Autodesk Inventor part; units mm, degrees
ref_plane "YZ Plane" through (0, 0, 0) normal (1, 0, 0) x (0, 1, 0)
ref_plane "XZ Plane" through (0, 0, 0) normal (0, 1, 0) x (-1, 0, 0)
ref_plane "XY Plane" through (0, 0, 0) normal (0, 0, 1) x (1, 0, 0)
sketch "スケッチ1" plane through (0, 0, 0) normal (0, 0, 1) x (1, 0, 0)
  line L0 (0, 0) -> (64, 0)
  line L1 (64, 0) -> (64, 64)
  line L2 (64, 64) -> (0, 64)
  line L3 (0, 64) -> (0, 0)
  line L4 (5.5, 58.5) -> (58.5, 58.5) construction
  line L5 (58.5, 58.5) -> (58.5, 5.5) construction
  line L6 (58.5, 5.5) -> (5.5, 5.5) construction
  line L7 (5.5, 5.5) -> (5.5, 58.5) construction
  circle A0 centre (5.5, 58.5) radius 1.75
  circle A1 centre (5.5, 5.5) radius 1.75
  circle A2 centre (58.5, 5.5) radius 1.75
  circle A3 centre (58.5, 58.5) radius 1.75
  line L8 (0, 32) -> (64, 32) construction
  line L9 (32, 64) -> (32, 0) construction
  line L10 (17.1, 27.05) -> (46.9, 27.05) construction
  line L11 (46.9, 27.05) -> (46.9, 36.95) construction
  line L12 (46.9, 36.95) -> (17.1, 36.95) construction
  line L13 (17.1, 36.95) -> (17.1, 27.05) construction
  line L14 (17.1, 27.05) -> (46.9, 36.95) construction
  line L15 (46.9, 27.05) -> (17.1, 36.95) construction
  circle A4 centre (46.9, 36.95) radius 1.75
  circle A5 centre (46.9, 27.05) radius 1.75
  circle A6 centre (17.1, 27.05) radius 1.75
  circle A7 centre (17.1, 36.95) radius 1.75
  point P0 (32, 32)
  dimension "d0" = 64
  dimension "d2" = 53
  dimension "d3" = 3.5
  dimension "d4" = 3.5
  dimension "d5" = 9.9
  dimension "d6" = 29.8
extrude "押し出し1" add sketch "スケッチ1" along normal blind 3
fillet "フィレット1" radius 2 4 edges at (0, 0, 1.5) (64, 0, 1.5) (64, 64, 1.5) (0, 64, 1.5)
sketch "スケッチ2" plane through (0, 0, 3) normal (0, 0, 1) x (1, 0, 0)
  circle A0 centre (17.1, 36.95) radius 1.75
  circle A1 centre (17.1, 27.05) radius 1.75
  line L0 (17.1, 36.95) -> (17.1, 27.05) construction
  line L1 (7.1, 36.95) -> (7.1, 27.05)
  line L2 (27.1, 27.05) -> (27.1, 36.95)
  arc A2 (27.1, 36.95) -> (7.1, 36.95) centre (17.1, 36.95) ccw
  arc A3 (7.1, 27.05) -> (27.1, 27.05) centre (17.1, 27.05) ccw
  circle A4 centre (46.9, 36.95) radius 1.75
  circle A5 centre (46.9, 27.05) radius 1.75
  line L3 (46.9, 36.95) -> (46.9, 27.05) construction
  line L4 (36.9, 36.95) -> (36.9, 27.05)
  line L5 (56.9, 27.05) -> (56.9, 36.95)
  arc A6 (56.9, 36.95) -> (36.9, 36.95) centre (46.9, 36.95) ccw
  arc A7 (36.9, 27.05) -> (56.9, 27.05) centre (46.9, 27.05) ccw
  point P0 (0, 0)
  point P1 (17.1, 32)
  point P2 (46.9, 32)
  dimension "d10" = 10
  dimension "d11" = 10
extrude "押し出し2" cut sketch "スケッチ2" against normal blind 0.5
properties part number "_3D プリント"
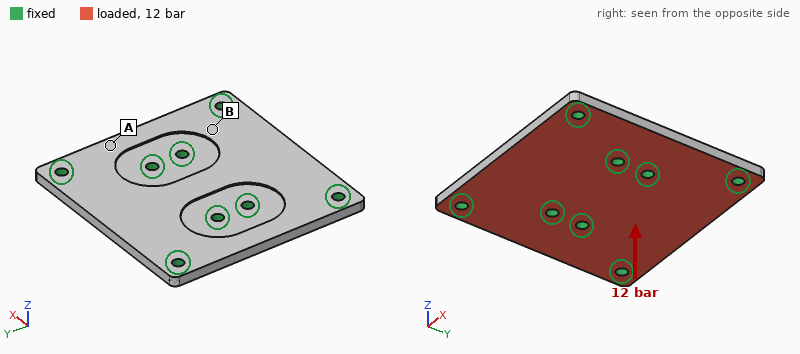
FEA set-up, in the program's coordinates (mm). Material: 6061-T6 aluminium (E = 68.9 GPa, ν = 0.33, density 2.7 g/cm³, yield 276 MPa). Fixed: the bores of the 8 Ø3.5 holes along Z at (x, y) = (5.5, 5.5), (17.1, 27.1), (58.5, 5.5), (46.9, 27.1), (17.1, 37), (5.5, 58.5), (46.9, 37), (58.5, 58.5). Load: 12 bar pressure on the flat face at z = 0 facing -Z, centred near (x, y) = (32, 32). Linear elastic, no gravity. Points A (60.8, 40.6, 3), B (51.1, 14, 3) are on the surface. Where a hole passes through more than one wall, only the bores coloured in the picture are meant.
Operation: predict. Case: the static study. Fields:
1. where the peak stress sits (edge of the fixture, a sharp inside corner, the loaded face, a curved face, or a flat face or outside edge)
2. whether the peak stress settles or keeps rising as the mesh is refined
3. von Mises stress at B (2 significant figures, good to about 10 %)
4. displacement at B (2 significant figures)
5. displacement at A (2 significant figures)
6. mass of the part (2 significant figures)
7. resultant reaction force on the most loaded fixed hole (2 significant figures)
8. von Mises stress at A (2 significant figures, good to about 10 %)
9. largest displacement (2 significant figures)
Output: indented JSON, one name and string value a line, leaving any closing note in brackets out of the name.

{
  "where the peak stress sits": "edge of the fixture",
  "whether the peak stress settles or keeps rising as the mesh is refined": "keeps rising",
  "von Mises stress at B": "61 MPa",
  "displacement at B": "0.021 mm",
  "displacement at A": "0.024 mm",
  "mass of the part": "31 g",
  "resultant reaction force on the most loaded fixed hole": "630 N",
  "von Mises stress at A": "27 MPa",
  "largest displacement": "0.13 mm"
}
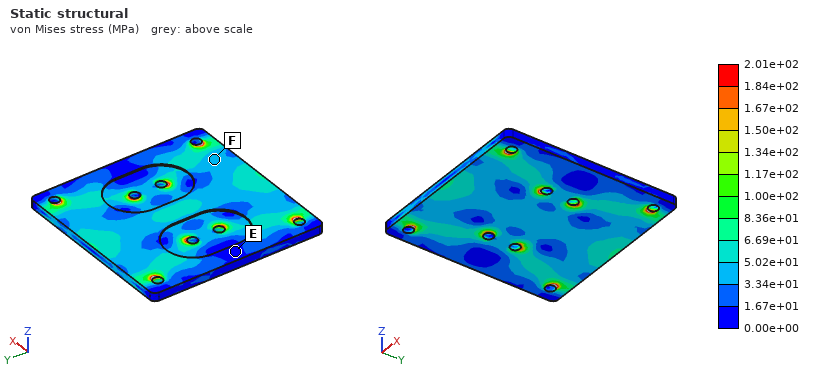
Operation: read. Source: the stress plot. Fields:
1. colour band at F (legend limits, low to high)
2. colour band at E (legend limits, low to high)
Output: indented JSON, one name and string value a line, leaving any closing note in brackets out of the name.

{
  "colour band at F": "3.34e+01 to 5.02e+01 MPa",
  "colour band at E": "0.00e+00 to 1.67e+01 MPa"
}
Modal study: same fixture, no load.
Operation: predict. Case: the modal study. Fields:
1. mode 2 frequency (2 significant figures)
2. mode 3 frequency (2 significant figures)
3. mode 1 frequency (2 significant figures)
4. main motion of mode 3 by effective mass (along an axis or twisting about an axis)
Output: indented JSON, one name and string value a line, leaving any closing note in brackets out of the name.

{
  "mode 2 frequency": "7000 Hz",
  "mode 3 frequency": "11 kHz",
  "mode 1 frequency": "6900 Hz",
  "main motion of mode 3 by effective mass": "twisting about Y"
}
